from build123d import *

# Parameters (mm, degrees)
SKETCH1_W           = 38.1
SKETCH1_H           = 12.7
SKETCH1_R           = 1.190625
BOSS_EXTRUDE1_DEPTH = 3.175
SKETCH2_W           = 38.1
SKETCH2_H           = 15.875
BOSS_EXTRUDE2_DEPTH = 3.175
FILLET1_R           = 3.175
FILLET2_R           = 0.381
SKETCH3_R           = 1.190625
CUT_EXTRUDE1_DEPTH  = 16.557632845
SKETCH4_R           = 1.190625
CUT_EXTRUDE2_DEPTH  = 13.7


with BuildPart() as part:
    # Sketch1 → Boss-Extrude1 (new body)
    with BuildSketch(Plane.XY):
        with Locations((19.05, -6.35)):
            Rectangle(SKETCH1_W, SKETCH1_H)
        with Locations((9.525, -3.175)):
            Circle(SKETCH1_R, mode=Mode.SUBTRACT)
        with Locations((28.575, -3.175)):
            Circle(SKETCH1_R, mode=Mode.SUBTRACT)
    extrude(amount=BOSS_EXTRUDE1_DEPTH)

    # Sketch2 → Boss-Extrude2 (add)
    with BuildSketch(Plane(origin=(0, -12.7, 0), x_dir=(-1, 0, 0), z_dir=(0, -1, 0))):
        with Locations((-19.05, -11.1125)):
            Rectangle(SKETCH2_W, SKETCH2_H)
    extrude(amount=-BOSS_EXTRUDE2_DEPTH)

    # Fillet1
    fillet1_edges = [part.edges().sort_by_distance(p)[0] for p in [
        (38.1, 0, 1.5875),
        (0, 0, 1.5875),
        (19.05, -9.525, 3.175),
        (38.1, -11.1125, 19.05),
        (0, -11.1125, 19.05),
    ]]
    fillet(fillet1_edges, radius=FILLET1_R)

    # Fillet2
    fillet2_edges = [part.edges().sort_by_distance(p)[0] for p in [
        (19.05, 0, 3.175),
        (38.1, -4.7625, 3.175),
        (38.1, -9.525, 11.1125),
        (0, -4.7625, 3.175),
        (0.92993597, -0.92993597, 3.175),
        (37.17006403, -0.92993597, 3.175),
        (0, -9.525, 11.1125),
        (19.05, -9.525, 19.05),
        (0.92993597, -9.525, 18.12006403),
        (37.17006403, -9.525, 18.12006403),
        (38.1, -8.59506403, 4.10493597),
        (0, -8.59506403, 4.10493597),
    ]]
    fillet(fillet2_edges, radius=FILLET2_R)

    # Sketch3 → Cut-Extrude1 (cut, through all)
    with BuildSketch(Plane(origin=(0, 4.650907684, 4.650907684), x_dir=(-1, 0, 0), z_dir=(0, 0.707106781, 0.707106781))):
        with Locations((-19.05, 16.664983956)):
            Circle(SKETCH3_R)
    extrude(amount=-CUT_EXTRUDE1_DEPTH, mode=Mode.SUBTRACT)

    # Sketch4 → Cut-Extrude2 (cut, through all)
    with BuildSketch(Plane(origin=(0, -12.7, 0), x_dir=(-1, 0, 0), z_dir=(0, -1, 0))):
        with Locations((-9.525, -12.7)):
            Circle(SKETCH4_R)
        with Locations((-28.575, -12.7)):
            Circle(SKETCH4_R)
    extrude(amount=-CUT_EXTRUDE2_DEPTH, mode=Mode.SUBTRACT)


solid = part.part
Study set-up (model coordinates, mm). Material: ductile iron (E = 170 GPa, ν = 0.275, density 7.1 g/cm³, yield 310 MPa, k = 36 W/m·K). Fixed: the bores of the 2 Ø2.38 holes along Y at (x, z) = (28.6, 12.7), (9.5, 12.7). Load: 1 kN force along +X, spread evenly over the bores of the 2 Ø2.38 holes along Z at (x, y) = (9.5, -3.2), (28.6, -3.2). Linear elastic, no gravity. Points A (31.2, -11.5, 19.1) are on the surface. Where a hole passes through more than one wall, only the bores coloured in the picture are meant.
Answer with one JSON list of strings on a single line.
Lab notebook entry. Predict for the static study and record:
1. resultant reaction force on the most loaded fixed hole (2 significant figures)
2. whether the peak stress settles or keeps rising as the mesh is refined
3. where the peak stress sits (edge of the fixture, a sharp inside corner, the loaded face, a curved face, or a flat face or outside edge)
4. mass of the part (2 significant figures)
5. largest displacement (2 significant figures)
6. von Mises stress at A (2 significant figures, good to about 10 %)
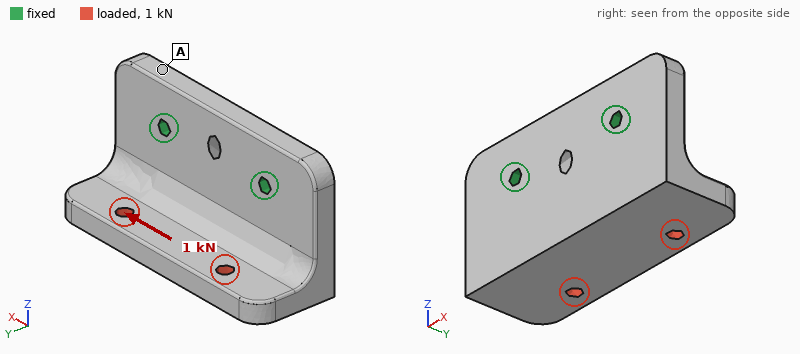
["800 N", "keeps rising", "edge of the fixture", "24 g", "25 µm", "22 MPa"]
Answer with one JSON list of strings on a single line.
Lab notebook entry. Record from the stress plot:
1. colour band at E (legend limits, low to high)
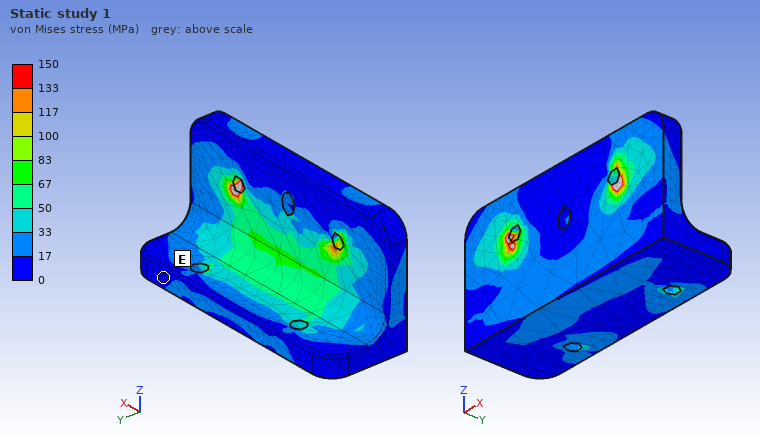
["0 to 17 MPa"]
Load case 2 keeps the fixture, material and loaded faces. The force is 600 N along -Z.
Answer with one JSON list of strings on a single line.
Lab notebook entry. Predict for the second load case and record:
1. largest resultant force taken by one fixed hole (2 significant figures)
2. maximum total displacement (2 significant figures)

["300 N", "45 µm"]
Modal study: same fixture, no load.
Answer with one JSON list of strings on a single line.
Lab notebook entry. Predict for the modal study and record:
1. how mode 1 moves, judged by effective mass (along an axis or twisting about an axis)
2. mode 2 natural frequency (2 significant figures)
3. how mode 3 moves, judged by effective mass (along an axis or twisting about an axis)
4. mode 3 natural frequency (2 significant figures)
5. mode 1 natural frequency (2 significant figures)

["along Y", "9400 Hz", "along X", "20 kHz", "6200 Hz"]
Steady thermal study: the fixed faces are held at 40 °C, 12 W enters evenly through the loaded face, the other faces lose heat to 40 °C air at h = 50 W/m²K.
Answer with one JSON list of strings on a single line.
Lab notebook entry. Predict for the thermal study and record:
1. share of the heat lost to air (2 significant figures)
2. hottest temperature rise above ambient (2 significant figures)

["23 %", "57 K"]
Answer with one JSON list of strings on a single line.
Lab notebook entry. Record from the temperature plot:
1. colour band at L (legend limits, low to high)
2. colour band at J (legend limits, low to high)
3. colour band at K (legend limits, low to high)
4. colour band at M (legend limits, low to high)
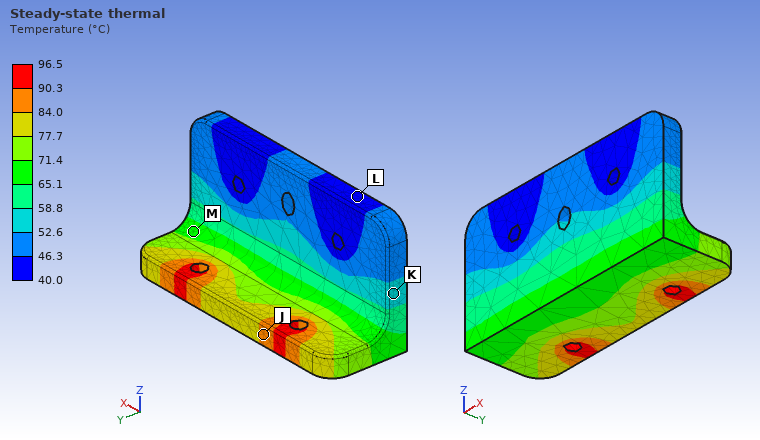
["40.0 to 46.3 °C", "84.0 to 90.3 °C", "52.6 to 58.8 °C", "65.1 to 71.4 °C"]
